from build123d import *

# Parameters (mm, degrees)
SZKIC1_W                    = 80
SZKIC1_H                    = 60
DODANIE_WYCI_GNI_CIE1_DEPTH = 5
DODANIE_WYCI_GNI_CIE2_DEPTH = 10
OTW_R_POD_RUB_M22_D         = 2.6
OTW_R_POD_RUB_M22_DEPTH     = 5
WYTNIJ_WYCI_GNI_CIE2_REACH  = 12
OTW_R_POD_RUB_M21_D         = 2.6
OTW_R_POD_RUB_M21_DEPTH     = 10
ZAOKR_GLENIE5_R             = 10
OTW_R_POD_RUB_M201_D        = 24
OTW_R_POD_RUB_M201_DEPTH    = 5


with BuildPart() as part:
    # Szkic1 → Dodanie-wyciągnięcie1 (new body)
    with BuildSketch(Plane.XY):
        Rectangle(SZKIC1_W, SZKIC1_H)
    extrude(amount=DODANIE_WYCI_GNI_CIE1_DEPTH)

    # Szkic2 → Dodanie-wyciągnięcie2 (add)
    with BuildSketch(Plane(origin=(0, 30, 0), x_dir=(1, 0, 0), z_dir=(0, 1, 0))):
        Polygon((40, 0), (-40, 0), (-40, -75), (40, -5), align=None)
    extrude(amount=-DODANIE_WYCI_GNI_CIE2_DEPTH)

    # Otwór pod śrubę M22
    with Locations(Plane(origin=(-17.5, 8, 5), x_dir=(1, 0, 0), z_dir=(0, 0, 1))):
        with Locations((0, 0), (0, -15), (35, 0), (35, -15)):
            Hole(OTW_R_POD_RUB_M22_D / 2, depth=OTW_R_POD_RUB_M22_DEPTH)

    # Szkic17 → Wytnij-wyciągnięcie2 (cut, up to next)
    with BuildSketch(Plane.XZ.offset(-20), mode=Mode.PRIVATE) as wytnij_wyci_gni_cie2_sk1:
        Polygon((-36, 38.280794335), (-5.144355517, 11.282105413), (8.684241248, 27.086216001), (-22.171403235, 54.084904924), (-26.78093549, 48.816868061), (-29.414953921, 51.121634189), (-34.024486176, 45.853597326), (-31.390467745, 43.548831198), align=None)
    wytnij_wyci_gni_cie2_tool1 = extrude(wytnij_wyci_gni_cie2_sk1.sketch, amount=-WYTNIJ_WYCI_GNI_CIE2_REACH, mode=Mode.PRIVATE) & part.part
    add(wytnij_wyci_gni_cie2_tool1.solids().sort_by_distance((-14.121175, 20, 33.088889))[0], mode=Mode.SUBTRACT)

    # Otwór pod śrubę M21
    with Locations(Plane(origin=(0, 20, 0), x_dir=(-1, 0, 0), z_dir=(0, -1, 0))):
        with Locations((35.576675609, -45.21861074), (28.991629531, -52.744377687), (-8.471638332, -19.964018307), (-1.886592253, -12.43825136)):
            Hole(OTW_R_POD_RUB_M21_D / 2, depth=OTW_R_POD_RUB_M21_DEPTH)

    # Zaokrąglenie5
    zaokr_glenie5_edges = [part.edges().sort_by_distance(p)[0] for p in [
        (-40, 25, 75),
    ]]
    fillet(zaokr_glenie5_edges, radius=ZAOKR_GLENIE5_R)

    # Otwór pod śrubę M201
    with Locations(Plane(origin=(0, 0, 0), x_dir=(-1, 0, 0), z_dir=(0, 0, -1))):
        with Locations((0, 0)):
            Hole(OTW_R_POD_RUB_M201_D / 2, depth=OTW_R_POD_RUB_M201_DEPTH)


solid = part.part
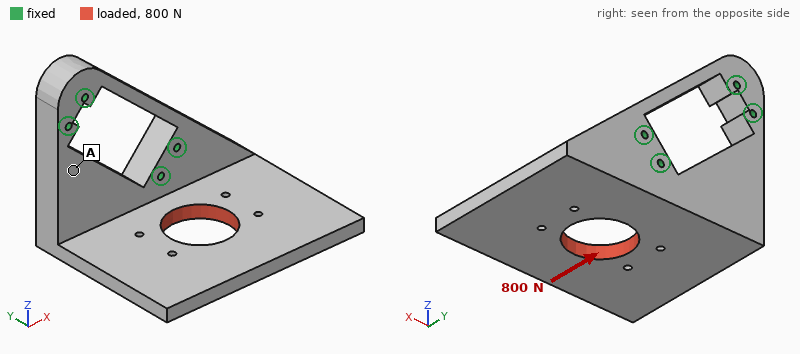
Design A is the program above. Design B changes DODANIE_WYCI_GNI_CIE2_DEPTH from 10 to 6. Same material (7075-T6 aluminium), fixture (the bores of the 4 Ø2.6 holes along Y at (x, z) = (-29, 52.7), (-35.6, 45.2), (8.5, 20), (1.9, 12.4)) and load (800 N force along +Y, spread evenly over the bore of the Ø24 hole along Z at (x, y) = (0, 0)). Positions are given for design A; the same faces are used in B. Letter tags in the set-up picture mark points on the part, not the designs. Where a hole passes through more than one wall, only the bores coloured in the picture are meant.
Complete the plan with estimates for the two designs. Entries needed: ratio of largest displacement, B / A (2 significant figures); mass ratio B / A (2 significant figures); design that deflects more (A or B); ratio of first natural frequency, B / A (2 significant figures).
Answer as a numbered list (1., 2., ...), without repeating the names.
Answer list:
1. 3.1
2. 0.82
3. B
4. 0.74
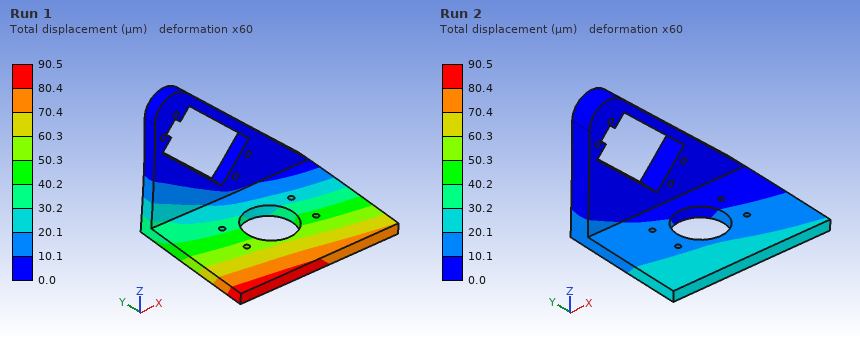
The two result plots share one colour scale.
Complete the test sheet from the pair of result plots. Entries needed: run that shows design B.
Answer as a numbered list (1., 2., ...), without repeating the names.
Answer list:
1. Run 1
